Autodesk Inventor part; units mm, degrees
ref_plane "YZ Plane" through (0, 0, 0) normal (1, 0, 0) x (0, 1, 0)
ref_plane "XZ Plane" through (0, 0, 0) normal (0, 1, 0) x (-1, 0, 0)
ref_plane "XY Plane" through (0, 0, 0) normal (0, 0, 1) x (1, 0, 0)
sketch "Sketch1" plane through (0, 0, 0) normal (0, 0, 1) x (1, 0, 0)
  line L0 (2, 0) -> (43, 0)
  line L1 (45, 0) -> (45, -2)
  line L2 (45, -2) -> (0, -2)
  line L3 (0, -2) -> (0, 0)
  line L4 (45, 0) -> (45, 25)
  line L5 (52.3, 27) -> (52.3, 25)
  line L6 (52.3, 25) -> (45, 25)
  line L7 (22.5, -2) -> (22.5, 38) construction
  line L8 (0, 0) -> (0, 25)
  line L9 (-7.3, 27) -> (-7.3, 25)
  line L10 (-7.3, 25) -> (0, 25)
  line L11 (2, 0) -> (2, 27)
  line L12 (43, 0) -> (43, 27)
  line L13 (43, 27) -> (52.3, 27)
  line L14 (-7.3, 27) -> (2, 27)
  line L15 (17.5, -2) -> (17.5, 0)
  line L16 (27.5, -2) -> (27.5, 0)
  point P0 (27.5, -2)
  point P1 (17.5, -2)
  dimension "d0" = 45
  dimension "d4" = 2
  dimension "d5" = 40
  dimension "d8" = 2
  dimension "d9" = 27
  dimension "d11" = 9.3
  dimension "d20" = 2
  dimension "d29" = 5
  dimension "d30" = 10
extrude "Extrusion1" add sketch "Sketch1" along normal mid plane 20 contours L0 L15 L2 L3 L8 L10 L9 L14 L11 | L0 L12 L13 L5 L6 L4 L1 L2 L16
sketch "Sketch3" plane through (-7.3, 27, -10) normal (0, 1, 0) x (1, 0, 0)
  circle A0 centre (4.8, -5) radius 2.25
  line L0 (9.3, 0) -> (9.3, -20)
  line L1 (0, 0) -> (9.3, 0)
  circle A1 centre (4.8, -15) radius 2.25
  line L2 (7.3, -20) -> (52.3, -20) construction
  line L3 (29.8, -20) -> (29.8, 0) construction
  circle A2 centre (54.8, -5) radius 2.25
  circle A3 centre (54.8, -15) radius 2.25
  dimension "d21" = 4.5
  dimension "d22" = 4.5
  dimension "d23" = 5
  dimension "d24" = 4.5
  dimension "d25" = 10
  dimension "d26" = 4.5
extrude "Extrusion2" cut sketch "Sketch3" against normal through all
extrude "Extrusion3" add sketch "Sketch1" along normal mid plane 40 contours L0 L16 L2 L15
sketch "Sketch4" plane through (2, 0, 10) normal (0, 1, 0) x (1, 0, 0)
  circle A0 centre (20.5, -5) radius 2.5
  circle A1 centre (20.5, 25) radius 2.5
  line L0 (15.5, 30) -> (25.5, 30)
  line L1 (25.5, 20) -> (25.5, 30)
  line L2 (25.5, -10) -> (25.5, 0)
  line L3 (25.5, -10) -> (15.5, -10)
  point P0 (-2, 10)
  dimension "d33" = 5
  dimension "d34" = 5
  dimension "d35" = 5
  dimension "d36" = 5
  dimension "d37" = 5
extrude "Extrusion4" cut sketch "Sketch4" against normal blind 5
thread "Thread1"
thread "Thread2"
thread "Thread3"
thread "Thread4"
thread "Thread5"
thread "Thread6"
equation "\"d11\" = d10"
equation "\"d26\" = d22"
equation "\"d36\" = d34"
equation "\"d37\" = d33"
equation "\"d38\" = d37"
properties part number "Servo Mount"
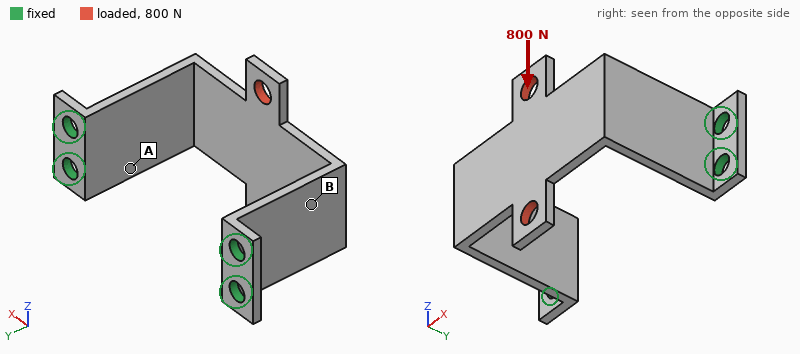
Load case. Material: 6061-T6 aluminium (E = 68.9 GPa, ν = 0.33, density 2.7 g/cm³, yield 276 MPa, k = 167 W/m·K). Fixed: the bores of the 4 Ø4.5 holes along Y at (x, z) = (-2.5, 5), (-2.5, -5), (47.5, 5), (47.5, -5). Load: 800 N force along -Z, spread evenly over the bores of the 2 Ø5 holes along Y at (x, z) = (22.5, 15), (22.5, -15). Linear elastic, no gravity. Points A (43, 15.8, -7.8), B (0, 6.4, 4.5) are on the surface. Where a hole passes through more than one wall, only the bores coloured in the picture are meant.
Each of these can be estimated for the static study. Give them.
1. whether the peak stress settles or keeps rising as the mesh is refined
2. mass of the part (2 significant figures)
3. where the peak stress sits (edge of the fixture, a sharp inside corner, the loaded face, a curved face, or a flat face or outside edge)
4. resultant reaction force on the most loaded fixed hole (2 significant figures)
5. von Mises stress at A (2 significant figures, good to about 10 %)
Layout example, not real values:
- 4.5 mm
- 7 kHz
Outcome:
- keeps rising
- 13 g
- edge of the fixture
- 910 N
- 32 MPa
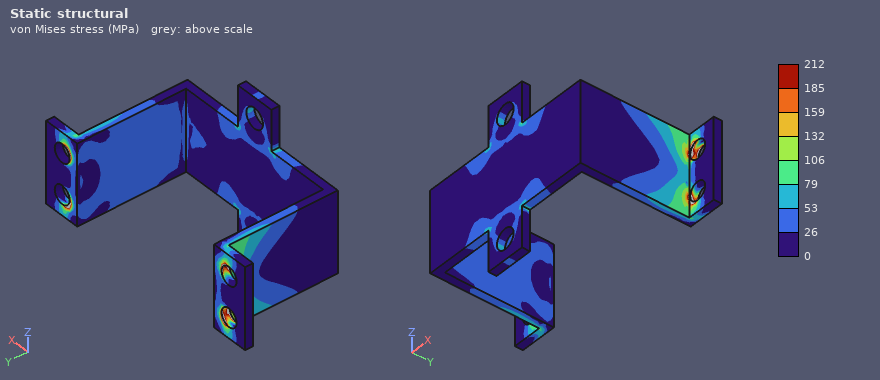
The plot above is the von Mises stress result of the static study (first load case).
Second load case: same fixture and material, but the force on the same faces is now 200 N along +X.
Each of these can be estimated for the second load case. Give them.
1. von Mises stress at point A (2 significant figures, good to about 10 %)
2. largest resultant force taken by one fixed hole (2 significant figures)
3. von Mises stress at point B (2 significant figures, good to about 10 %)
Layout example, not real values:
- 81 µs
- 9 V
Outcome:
- 38 MPa
- 58 N
- 26 MPa
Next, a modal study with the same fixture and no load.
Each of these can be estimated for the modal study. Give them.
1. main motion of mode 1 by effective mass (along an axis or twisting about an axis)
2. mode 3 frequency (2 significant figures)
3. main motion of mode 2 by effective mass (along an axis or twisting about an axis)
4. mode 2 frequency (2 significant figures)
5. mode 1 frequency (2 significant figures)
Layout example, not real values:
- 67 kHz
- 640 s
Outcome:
- along X
- 4000 Hz
- along Y
- 3300 Hz
- 1500 Hz
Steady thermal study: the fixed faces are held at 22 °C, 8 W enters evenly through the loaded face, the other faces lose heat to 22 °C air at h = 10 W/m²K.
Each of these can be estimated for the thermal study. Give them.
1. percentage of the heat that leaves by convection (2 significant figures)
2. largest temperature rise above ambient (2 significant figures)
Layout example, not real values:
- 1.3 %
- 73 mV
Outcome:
- 9.1 %
- 38 K
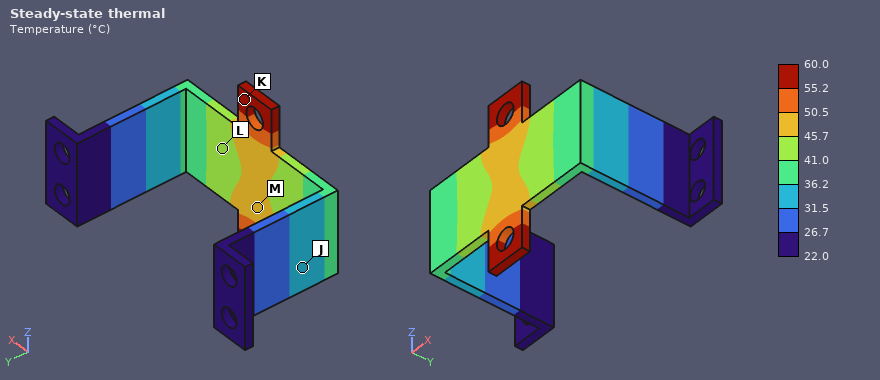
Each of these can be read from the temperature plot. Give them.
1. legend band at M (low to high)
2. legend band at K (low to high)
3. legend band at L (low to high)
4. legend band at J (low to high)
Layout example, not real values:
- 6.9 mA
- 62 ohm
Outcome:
- 45.7 to 50.5 °C
- 55.2 to 60.0 °C
- 41.0 to 45.7 °C
- 31.5 to 36.2 °C
